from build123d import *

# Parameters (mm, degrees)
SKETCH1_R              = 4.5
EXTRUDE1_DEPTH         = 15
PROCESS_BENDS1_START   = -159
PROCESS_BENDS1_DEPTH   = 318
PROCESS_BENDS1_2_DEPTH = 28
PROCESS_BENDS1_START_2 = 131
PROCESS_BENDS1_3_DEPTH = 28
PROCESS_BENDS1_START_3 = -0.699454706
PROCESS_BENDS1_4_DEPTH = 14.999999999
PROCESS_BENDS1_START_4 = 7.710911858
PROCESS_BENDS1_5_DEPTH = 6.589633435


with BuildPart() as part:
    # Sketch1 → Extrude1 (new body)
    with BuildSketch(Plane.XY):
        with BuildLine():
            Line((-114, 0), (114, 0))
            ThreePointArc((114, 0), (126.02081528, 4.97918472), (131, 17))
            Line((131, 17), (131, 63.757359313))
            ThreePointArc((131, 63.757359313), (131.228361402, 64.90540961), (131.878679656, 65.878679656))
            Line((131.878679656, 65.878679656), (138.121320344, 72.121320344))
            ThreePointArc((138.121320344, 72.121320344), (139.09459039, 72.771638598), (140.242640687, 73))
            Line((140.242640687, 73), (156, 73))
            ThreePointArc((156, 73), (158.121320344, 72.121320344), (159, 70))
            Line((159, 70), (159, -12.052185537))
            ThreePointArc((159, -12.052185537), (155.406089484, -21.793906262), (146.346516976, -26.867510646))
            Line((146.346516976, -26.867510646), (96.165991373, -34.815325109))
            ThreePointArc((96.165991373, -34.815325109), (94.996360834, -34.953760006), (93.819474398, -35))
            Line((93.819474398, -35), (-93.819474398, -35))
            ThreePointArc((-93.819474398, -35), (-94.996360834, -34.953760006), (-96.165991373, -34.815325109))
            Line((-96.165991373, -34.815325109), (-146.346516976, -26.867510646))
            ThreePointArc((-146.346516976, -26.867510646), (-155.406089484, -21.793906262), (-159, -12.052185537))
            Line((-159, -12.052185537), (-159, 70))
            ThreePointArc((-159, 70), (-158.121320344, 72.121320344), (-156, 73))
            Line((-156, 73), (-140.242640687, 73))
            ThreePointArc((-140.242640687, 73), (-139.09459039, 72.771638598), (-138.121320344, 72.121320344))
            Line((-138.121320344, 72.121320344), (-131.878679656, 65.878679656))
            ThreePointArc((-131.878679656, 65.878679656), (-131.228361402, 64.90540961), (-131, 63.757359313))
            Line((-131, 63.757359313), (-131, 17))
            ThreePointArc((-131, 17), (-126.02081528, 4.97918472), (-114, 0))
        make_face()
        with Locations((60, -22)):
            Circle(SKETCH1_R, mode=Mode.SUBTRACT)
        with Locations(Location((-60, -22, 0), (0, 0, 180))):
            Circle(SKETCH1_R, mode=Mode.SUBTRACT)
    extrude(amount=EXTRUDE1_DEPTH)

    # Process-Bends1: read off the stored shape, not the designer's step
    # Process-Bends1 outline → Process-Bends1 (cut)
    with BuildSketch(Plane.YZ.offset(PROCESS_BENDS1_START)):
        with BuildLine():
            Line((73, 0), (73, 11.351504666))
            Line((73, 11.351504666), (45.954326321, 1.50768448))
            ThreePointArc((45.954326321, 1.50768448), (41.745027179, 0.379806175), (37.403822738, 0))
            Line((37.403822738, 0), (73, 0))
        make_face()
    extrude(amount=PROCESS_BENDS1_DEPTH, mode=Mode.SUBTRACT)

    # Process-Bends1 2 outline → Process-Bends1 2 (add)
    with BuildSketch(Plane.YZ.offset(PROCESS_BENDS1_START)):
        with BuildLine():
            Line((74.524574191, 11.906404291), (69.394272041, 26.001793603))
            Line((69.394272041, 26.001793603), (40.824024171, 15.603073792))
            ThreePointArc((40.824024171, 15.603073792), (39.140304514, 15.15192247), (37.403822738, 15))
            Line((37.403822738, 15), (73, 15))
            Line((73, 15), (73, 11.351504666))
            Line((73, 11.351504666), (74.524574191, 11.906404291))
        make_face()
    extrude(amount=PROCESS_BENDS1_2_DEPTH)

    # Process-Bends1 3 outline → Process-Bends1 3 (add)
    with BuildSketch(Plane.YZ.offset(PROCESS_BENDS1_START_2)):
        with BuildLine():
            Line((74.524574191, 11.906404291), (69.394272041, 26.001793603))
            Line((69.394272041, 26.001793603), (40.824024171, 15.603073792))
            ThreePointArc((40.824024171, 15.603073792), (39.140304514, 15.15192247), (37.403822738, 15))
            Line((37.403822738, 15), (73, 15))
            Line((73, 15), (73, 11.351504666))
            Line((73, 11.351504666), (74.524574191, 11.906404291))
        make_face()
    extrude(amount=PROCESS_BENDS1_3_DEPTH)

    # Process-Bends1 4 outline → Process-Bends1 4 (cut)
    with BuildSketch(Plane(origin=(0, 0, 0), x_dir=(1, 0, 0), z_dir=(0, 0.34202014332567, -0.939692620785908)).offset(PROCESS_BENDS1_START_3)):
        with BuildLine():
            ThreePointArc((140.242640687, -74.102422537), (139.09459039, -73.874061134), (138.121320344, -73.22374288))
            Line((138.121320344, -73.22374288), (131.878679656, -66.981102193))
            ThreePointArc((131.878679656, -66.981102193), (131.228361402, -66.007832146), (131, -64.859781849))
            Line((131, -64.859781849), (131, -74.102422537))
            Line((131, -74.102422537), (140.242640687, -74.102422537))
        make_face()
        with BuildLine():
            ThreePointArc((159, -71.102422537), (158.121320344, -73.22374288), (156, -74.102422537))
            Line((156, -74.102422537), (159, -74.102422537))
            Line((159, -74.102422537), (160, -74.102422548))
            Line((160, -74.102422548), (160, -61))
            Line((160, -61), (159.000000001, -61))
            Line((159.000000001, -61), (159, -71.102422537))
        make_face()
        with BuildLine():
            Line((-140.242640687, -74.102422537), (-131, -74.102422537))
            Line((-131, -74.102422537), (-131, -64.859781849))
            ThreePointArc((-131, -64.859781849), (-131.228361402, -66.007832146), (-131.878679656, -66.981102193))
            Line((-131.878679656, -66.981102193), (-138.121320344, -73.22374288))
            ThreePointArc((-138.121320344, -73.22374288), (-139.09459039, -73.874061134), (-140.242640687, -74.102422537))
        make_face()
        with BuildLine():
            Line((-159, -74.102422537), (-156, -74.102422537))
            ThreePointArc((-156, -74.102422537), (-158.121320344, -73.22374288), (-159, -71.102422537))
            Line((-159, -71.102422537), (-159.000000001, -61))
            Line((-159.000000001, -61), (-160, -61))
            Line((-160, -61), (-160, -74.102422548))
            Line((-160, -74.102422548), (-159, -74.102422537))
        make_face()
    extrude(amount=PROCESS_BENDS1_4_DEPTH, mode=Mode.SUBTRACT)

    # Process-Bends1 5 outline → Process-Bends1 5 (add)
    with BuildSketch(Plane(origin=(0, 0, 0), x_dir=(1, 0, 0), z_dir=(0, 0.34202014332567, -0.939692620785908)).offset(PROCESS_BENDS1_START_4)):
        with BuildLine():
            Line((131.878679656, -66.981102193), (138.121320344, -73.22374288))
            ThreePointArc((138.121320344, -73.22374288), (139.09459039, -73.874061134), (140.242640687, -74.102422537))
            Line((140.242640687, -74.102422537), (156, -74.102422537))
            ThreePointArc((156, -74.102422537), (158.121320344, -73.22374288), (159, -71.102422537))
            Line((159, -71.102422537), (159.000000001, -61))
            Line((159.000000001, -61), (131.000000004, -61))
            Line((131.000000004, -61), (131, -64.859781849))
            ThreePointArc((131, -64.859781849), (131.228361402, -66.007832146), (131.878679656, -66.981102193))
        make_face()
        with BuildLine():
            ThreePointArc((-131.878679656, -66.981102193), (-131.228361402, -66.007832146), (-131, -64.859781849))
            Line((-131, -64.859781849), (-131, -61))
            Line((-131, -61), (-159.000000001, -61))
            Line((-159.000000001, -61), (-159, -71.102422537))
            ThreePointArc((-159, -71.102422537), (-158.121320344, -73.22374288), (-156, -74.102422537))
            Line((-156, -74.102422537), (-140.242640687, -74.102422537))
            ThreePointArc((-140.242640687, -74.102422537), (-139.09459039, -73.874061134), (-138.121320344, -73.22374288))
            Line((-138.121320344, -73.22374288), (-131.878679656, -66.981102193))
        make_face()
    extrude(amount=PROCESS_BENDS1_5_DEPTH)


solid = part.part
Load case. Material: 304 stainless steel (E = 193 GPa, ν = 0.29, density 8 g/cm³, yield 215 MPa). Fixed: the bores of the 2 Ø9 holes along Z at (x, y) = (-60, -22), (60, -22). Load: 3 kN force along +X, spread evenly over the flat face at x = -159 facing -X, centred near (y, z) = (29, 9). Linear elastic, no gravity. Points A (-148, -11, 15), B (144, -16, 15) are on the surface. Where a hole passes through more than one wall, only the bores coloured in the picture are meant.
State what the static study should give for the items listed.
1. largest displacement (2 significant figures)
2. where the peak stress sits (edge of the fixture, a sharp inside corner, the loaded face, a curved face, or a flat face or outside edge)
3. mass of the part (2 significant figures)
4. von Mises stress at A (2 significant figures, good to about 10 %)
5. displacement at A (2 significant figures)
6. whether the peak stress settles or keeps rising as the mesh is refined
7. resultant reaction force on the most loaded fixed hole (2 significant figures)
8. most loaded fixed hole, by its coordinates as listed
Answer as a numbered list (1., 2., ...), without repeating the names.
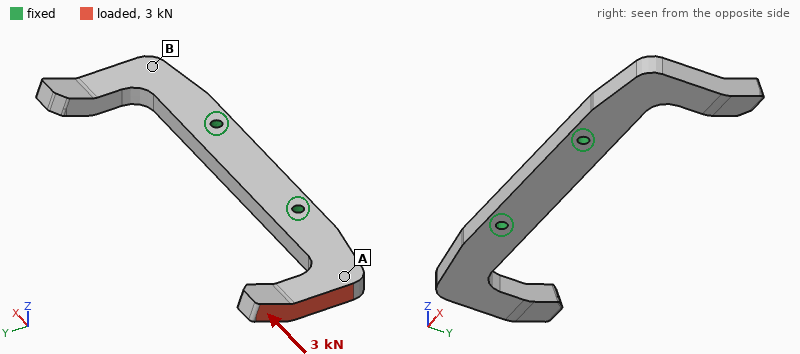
1. 0.19 mm
2. edge of the fixture
3. 1.7 kg
4. 17 MPa
5. 0.080 mm
6. keeps rising
7. 1.8 kN
8. (-60, -22)
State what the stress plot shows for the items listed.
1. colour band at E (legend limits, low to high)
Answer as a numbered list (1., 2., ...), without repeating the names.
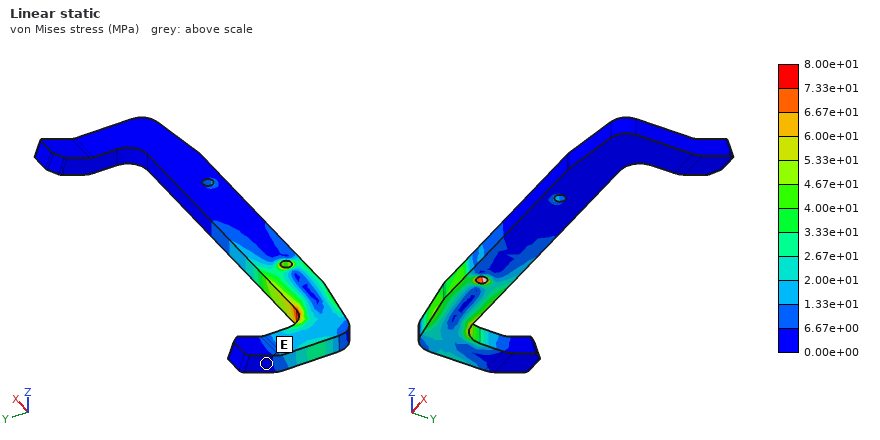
1. 0.00e+00 to 6.67e+00 MPa
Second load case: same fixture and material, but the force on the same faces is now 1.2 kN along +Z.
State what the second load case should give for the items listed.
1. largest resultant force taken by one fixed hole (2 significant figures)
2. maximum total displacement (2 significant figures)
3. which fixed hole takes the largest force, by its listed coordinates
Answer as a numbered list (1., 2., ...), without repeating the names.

1. 1.3 kN
2. 0.45 mm
3. (-60, -22)
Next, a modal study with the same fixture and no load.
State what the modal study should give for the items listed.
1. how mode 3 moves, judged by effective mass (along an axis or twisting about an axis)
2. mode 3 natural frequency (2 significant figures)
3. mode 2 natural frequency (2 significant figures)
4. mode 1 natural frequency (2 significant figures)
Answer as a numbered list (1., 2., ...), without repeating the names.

1. along Y
2. 1100 Hz
3. 600 Hz
4. 600 Hz
